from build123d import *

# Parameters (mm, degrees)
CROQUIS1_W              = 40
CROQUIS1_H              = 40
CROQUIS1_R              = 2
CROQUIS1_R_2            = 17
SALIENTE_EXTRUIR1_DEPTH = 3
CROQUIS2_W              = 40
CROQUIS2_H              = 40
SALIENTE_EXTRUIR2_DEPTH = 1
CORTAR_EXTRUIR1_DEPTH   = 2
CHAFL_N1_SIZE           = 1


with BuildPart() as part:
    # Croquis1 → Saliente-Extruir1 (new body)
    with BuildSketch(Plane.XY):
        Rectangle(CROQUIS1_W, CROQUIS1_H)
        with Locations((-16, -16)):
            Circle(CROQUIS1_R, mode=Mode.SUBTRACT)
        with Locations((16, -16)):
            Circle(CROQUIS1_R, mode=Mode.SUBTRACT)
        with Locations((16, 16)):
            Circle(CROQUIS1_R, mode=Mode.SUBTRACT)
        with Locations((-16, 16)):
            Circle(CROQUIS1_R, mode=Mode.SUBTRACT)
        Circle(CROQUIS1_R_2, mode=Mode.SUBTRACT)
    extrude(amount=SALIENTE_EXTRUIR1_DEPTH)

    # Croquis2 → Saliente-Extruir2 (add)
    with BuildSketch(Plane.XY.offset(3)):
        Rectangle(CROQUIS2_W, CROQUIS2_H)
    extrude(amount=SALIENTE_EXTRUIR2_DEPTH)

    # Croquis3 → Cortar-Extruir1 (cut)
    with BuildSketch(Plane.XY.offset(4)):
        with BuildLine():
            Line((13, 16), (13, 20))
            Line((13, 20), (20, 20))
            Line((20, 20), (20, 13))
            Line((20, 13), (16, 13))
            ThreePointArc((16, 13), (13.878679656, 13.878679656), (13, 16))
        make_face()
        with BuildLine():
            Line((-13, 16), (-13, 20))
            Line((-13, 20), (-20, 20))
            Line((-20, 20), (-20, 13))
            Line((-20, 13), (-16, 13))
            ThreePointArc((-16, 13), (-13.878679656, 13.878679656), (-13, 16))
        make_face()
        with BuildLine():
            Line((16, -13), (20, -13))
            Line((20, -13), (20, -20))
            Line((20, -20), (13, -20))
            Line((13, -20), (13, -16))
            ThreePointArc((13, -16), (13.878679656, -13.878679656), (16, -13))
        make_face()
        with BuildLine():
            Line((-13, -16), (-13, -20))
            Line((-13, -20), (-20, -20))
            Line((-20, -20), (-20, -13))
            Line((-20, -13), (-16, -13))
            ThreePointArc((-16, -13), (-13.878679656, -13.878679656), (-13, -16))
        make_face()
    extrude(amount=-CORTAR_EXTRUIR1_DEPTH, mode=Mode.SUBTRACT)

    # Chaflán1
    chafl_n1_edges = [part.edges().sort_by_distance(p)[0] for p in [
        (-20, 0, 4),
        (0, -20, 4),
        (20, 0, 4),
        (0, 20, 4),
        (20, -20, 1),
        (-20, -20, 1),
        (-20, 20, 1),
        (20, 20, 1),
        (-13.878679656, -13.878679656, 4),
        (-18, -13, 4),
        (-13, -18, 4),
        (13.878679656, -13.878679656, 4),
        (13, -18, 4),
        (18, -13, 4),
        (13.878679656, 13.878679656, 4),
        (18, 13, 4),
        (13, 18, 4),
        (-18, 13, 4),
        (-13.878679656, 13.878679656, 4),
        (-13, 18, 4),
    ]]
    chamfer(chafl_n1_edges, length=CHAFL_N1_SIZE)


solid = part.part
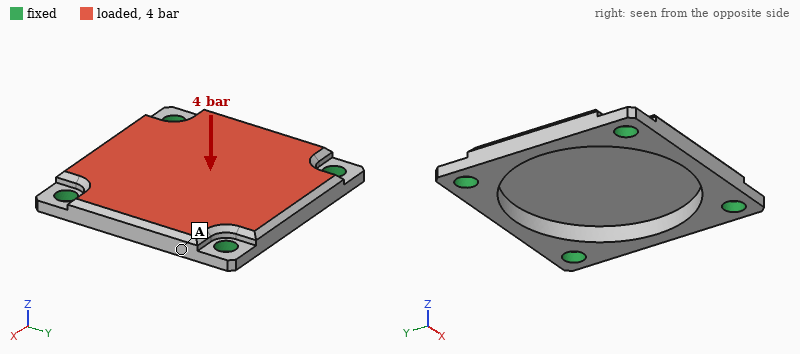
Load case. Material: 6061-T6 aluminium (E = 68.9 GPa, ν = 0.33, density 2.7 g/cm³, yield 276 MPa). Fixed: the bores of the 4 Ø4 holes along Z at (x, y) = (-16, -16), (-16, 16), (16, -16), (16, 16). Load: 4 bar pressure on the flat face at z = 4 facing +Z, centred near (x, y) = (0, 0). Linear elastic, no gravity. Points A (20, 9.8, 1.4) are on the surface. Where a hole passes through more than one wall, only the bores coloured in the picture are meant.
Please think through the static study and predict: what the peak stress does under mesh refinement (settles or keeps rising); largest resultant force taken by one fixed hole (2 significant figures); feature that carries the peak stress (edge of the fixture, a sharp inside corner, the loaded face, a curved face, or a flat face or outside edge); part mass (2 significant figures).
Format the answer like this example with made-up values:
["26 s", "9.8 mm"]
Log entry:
["keeps rising", "230 N", "edge of the fixture", "8.4 g"]
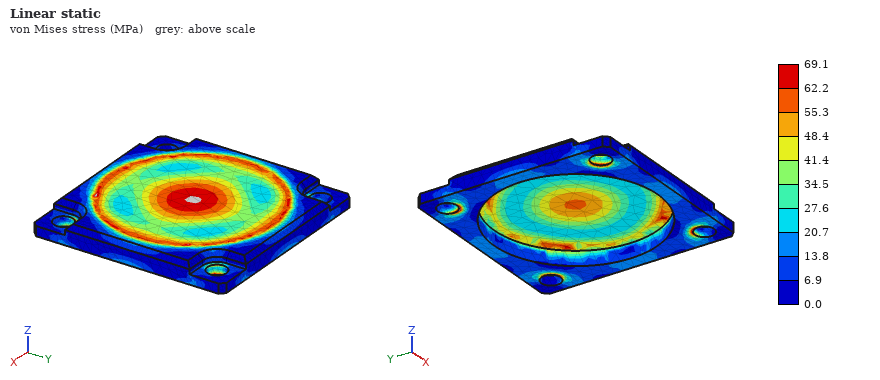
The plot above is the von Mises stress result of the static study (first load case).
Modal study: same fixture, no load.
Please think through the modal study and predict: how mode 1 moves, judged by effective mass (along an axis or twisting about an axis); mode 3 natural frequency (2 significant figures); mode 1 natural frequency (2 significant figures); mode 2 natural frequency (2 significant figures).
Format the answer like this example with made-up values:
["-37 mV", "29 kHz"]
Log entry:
["along Z", "15 kHz", "7700 Hz", "15 kHz"]
